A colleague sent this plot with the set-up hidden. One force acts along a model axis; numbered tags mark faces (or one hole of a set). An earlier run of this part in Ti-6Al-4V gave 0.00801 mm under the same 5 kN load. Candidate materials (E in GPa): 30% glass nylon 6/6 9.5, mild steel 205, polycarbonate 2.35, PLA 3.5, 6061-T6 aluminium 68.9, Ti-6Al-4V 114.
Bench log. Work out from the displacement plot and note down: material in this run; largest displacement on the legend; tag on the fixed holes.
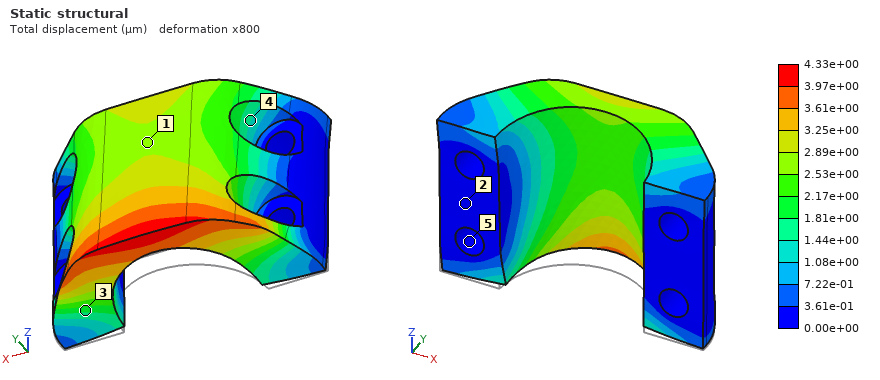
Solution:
mild steel
4.33e+00 µm
5
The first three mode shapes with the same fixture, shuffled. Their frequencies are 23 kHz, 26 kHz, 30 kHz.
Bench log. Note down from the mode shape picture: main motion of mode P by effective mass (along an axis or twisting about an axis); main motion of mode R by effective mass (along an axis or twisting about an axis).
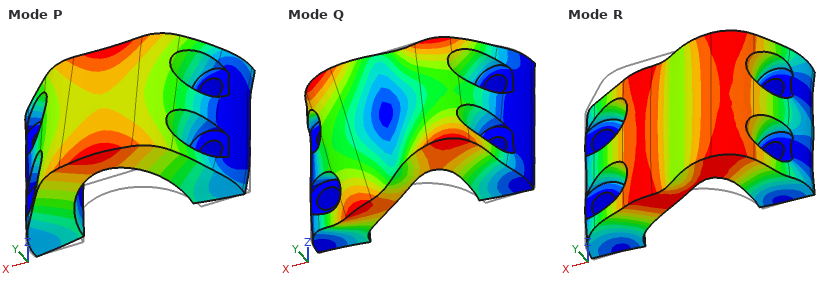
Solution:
along Z
along X
